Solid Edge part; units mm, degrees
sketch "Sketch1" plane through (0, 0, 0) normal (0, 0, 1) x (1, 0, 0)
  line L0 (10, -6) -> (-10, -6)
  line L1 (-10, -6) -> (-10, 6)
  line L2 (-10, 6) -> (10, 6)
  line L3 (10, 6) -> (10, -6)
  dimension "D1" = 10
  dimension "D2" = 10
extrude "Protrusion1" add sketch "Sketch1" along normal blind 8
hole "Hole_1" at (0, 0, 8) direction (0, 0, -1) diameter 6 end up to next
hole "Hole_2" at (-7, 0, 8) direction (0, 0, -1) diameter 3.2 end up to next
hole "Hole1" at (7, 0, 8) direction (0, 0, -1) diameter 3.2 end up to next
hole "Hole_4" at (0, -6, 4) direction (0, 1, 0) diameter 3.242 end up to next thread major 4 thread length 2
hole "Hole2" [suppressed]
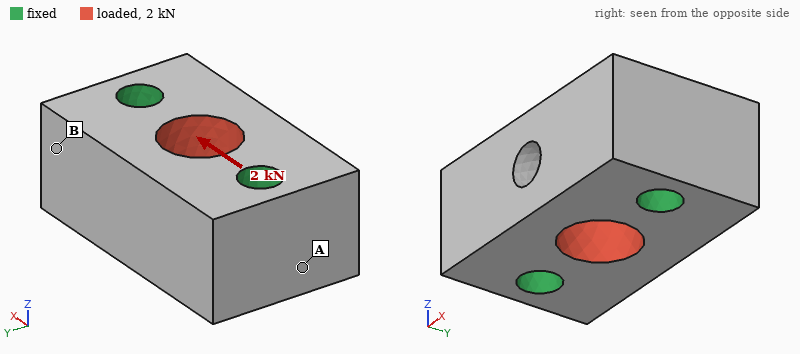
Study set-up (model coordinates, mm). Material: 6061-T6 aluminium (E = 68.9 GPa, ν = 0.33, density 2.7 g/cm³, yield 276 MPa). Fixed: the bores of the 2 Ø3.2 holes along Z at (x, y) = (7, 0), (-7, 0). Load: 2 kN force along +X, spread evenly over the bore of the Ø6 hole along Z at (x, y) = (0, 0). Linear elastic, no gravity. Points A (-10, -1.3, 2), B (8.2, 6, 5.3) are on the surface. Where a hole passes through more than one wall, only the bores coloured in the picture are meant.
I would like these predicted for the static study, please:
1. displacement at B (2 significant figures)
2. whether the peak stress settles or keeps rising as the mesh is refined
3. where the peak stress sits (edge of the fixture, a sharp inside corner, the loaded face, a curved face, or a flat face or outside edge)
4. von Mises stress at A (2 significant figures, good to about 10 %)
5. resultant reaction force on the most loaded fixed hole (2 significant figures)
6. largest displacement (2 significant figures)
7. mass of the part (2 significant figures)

1.1 µm
keeps rising
edge of the fixture
7.9 MPa
1.0 kN
1.8 µm
4.2 g
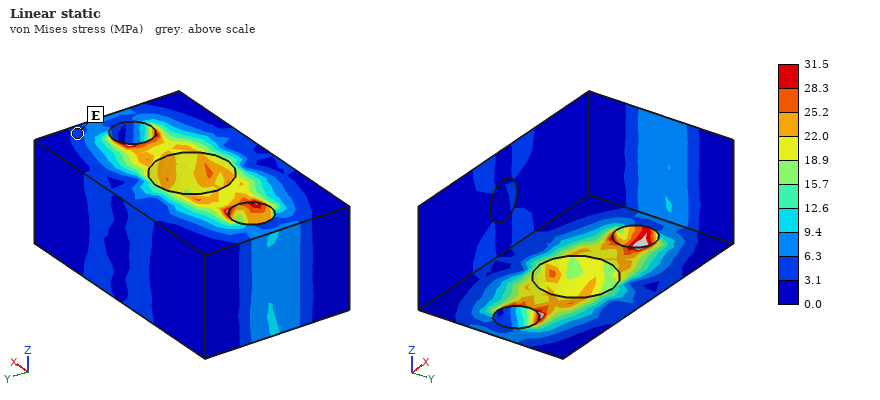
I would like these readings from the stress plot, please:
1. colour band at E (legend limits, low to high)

3.1 to 6.3 MPa
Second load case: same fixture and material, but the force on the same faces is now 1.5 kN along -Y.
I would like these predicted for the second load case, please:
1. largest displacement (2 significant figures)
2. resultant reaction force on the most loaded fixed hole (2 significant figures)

2.7 µm
750 N
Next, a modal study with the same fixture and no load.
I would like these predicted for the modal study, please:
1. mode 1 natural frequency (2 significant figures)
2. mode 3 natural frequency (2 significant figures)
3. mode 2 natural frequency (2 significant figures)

87 kHz
95 kHz
93 kHz
